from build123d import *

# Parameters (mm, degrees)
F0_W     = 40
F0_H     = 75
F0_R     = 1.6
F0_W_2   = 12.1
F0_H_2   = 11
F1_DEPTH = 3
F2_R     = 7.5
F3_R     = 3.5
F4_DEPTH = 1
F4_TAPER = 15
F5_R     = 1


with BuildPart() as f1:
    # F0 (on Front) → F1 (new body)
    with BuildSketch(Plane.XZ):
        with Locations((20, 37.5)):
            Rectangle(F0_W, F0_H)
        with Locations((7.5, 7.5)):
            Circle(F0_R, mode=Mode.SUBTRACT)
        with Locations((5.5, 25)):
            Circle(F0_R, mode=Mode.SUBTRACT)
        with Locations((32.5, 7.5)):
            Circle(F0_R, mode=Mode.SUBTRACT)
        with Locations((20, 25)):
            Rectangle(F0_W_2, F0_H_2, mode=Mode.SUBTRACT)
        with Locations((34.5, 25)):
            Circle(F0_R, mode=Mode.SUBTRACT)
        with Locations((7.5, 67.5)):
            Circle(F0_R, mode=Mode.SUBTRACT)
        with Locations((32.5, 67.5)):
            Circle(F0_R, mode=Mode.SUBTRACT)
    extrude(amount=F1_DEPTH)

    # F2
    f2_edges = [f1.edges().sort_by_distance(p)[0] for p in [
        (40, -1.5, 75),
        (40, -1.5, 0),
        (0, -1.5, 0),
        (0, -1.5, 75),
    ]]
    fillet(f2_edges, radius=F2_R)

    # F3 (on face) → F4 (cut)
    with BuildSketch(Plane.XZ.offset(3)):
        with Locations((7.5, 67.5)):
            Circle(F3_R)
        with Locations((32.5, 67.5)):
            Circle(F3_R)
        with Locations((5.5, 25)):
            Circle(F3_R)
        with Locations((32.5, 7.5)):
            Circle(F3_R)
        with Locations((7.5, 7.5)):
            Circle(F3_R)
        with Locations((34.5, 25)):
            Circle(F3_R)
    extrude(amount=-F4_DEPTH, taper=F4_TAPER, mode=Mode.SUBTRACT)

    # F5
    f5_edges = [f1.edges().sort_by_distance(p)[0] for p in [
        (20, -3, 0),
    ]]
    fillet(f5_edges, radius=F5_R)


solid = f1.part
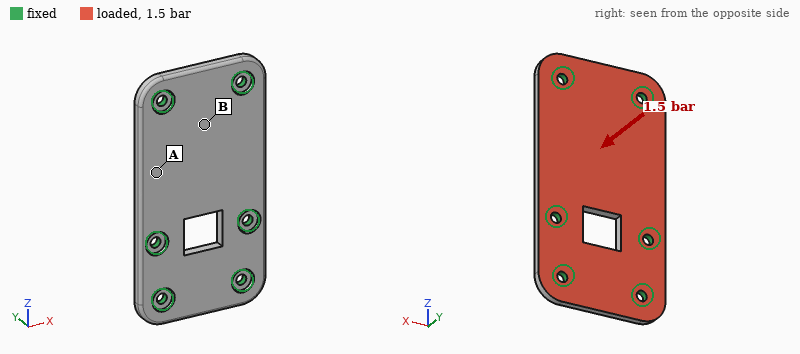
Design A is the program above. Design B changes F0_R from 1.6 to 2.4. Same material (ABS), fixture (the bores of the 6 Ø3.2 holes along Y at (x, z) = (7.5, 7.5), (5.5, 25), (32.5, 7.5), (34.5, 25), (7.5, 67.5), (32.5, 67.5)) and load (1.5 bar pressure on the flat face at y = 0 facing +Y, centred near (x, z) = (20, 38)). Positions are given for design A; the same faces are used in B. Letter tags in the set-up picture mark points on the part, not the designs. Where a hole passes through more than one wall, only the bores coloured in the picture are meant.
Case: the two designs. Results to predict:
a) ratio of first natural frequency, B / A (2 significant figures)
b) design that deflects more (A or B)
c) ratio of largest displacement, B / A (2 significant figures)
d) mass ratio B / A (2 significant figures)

1.1
A
0.80
0.99
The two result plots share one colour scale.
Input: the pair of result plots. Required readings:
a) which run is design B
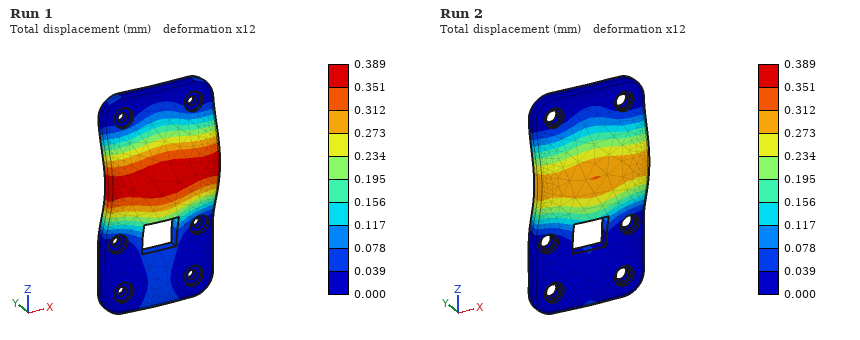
Run 2
